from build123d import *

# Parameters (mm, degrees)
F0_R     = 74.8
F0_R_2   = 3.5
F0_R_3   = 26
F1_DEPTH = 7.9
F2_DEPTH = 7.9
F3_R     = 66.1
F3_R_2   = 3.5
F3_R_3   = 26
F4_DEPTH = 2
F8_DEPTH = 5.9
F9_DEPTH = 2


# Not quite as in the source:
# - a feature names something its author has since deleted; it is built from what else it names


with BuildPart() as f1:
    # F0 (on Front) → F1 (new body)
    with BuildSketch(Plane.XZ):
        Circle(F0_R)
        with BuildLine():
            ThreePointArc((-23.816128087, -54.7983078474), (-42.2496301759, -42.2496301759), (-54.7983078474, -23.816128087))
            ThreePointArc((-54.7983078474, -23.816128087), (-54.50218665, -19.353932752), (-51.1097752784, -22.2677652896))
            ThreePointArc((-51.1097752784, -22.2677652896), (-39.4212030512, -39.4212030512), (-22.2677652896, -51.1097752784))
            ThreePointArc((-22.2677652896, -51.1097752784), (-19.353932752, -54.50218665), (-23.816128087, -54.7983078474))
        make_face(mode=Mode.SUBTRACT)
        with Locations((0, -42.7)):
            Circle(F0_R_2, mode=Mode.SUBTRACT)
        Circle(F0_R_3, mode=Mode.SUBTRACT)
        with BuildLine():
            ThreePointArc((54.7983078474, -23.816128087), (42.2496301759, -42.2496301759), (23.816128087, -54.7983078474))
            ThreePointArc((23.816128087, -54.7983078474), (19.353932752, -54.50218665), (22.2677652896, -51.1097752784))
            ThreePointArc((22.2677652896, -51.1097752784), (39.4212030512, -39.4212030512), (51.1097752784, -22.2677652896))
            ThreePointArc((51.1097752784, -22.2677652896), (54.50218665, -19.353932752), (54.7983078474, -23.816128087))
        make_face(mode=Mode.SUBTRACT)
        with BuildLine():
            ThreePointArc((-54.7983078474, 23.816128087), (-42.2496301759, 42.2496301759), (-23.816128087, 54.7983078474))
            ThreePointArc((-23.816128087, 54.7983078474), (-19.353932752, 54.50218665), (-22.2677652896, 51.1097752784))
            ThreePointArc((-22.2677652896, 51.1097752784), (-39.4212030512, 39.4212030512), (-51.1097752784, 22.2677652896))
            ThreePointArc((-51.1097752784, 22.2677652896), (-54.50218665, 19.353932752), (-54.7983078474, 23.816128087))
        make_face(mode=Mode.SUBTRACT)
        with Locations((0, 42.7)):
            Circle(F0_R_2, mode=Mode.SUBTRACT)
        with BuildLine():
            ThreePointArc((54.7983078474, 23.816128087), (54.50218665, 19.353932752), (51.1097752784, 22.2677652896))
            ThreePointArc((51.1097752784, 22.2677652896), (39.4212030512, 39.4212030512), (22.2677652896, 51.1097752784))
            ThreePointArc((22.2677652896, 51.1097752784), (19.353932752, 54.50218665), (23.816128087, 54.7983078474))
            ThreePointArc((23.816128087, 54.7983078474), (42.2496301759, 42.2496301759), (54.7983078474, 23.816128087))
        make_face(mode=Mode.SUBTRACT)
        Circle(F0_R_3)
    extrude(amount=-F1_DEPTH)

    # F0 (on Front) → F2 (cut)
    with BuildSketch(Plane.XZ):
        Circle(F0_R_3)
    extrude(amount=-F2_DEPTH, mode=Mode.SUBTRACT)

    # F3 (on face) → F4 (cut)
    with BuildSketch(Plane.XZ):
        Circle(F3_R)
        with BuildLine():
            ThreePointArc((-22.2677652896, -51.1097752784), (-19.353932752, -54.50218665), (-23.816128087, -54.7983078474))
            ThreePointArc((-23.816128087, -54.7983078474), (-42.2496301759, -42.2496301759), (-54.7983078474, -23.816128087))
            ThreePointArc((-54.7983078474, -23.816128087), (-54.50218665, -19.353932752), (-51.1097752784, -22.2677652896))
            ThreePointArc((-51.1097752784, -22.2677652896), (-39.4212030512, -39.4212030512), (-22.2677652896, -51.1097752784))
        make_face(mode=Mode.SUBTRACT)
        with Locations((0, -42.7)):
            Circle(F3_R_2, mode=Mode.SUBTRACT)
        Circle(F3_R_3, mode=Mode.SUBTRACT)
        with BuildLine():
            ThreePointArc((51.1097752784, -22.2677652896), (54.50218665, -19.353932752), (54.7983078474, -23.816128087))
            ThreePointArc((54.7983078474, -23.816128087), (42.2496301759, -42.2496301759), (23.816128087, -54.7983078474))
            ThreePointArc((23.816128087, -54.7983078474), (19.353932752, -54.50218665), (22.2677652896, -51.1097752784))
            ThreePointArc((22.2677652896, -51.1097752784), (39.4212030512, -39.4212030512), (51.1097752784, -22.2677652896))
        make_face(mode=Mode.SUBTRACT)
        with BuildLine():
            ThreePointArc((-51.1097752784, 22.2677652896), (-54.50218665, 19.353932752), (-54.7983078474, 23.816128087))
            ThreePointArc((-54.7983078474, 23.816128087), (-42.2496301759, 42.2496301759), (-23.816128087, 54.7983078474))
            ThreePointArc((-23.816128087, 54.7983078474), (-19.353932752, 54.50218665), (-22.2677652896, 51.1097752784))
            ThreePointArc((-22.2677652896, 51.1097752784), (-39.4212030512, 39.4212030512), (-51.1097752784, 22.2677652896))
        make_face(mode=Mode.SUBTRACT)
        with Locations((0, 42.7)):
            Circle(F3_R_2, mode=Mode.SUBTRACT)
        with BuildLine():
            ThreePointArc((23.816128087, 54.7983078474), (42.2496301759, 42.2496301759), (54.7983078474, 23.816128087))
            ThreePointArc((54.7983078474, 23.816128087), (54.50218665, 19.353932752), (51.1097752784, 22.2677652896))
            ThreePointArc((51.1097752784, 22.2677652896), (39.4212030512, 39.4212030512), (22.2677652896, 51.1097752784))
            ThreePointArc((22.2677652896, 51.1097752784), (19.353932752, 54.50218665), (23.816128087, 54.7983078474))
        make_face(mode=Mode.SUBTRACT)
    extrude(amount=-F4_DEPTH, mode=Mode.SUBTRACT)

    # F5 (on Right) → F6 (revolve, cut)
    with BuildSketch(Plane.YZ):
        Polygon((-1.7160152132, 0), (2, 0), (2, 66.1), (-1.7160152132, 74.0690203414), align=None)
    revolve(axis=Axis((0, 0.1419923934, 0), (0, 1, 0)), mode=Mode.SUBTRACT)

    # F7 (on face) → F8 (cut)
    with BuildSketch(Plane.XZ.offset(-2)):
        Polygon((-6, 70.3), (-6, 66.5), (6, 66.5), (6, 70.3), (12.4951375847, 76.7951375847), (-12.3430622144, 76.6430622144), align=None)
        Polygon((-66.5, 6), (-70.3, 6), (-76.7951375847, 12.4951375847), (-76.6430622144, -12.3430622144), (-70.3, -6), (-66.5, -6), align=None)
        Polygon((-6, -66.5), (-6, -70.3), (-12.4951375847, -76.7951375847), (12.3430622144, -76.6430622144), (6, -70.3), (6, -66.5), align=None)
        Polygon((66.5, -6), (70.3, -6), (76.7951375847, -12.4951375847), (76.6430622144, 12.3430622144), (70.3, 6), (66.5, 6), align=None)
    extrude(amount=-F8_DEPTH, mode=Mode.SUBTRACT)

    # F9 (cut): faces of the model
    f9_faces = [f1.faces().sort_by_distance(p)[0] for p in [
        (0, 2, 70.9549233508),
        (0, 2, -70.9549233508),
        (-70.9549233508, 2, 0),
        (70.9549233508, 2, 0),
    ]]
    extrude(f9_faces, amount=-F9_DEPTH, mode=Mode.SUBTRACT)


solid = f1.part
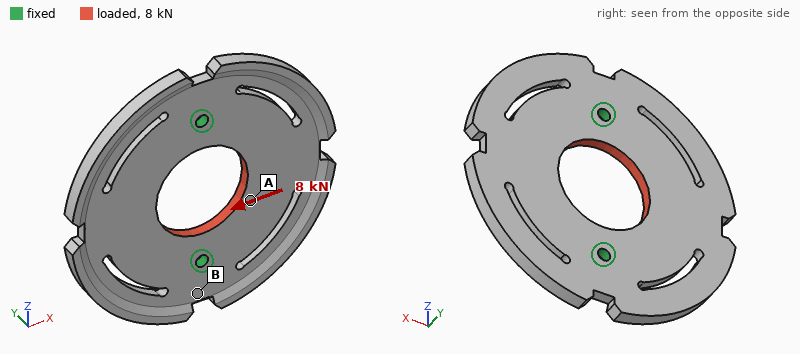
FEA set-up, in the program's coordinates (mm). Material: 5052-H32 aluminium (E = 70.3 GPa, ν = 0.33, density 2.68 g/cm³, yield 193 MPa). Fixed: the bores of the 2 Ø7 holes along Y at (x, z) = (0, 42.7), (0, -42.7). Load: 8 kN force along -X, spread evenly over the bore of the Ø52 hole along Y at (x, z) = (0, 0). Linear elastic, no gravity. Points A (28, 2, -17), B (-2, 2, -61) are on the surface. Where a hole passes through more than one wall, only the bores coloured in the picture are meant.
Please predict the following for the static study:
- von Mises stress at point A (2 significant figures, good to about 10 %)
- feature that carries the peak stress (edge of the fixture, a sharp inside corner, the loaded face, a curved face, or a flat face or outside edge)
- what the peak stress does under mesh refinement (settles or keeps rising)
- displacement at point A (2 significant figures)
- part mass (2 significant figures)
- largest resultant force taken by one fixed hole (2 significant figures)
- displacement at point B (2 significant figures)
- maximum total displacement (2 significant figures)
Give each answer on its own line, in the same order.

9.6 MPa
edge of the fixture
keeps rising
11 µm
240 g
4.0 kN
2.8 µm
14 µm
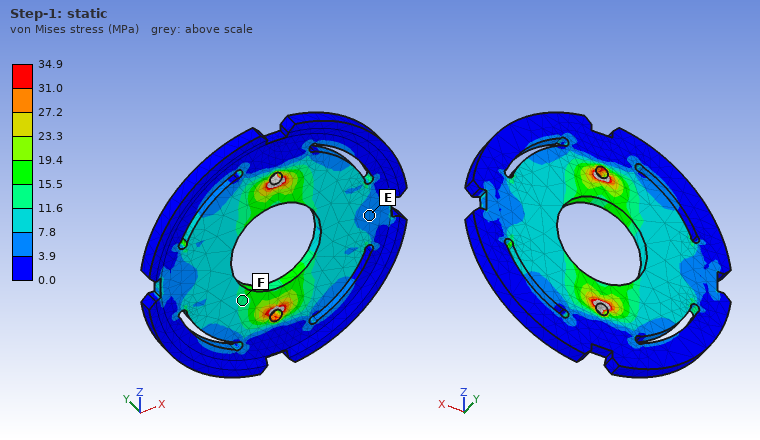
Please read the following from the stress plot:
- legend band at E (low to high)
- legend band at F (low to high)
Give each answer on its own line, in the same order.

3.9 to 7.8 MPa
11.6 to 15.5 MPa
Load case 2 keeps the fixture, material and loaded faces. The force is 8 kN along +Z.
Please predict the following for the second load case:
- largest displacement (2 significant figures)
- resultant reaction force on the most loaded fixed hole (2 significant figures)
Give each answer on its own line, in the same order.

15 µm
4.0 kN
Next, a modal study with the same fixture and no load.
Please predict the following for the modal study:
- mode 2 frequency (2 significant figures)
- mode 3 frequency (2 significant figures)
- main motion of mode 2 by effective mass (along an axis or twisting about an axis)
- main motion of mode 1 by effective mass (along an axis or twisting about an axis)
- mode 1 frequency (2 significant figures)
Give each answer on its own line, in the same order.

930 Hz
1800 Hz
along Y
twisting about Z
850 Hz
